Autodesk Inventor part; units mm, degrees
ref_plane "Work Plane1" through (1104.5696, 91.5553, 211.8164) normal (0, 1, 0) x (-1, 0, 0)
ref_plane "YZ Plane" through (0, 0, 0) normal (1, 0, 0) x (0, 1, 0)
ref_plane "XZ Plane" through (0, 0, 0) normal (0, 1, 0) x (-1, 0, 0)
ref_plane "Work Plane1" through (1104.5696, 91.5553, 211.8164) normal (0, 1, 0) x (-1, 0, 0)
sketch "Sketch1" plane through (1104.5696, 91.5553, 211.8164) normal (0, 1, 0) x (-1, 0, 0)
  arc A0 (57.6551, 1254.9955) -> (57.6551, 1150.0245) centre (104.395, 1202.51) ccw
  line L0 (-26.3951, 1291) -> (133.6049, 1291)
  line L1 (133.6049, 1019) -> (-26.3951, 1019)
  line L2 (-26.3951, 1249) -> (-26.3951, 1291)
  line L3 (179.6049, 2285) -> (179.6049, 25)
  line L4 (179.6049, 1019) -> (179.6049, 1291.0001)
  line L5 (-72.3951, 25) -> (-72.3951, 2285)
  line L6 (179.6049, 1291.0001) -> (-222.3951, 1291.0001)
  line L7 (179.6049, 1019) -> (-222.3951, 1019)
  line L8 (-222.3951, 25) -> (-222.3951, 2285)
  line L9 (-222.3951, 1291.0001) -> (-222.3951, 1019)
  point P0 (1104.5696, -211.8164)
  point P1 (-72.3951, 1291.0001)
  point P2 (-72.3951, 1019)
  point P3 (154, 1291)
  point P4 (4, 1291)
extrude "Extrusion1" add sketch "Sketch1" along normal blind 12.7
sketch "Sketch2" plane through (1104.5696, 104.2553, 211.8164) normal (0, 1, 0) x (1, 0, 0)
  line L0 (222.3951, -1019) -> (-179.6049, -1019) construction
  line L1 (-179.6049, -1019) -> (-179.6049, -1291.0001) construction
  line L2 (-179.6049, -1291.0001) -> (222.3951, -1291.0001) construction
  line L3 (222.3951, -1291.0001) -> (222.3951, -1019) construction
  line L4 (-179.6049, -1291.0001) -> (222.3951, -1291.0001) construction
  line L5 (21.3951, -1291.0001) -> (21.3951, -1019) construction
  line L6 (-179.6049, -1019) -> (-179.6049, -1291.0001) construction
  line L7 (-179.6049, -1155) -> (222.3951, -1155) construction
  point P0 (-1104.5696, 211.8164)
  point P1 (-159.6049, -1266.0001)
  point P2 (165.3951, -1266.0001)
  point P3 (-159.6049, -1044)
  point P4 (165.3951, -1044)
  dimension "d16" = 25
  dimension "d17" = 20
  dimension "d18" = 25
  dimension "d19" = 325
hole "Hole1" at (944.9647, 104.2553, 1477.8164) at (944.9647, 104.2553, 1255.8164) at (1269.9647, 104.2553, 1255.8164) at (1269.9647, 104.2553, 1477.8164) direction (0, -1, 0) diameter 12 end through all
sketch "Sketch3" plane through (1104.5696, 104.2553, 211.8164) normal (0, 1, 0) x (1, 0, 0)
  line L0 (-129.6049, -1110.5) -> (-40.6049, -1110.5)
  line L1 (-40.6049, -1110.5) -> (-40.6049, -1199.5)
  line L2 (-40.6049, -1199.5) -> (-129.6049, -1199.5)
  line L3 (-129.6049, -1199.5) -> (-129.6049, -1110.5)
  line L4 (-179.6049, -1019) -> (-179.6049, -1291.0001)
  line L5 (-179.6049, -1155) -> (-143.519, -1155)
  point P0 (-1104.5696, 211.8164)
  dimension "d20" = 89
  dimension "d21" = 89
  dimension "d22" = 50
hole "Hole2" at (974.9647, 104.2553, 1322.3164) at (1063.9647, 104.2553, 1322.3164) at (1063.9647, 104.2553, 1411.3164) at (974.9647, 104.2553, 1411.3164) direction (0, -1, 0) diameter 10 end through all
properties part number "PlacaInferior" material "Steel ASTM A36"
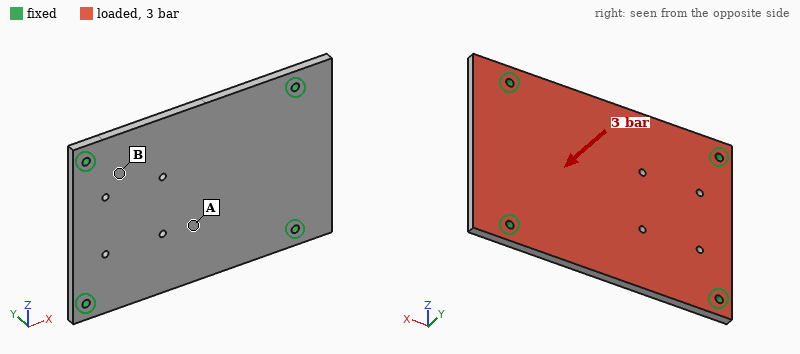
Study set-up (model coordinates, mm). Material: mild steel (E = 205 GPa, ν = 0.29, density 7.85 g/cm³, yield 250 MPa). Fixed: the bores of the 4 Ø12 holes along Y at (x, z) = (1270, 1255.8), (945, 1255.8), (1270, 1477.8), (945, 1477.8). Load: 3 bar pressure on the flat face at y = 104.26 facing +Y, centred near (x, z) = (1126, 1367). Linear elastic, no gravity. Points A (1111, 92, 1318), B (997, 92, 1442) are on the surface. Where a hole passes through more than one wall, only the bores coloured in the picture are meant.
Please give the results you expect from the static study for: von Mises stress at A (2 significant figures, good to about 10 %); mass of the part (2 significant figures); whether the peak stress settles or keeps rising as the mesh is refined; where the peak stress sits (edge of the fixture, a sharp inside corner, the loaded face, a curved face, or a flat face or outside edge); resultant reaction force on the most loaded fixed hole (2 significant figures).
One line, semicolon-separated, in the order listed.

52 MPa; 11 kg; keeps rising; edge of the fixture; 9.0 kN
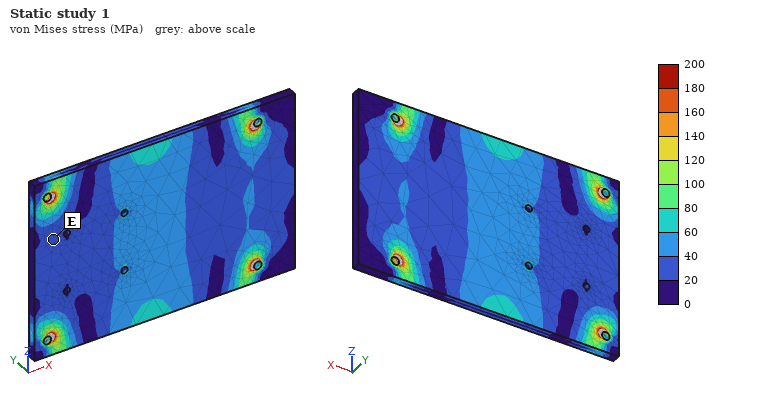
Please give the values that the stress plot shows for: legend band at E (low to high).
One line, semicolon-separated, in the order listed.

20 to 40 MPa
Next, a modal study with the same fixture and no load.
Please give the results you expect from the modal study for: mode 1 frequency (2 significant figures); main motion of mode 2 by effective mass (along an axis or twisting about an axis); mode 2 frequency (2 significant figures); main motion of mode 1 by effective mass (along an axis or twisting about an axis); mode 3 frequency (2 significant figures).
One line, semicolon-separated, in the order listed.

500 Hz; twisting about X; 780 Hz; along Y; 1100 Hz
